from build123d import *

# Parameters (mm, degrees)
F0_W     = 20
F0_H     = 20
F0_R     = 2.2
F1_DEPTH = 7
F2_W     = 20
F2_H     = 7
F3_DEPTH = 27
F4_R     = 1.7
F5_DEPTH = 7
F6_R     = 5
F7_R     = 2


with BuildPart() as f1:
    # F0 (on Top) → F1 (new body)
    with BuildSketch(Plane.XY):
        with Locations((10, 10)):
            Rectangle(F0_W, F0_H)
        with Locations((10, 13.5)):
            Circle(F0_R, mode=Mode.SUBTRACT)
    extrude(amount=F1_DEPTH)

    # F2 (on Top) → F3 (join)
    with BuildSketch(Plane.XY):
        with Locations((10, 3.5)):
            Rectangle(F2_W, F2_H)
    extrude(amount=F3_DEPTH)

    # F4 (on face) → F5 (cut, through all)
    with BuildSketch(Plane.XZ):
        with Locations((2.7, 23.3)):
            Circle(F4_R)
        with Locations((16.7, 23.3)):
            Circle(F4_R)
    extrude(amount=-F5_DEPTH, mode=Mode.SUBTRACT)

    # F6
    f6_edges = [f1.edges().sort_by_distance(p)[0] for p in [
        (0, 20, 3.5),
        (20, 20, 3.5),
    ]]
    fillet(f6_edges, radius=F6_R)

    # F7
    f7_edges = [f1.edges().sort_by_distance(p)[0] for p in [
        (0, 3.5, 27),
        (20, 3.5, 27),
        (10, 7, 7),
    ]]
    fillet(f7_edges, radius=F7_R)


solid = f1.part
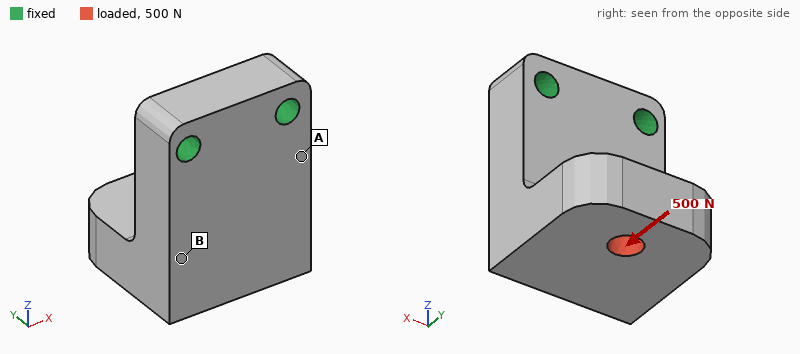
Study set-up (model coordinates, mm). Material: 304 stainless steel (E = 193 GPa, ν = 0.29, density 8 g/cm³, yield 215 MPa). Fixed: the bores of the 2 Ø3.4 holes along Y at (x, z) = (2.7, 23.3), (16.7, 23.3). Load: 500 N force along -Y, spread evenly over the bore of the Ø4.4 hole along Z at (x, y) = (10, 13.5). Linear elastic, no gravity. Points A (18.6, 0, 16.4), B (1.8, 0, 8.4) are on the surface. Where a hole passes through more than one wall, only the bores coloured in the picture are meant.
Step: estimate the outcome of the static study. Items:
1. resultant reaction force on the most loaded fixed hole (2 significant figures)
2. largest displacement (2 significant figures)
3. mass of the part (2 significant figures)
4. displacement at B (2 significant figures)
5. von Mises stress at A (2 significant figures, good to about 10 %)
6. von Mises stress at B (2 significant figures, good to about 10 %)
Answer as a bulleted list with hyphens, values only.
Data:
- 260 N
- 22 µm
- 42 g
- 8.7 µm
- 42 MPa
- 14 MPa
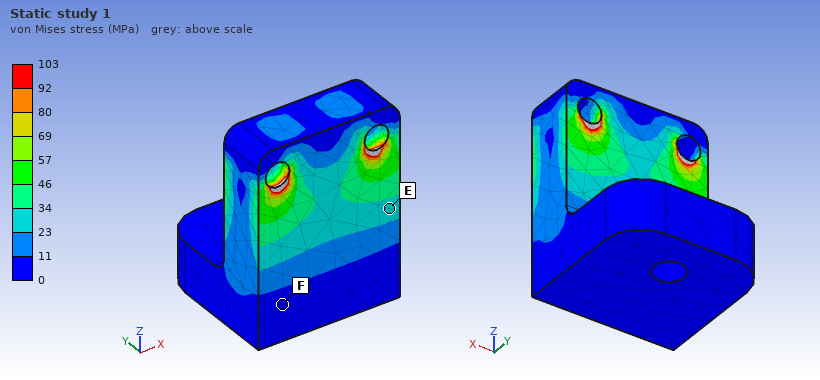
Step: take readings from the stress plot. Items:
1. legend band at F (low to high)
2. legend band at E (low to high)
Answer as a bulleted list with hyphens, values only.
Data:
- 0 to 11 MPa
- 23 to 34 MPa
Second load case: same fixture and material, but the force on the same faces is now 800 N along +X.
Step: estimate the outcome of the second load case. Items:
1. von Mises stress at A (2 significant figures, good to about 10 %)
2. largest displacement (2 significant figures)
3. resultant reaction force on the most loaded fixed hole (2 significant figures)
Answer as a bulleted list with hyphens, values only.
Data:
- 35 MPa
- 17 µm
- 1.2 kN
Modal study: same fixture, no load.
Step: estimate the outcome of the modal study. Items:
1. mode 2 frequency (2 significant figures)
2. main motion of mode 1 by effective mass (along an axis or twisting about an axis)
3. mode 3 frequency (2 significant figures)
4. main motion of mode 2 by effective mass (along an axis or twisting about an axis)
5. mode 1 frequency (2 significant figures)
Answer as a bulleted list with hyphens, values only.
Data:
- 9900 Hz
- along Y
- 18 kHz
- along X
- 5600 Hz
